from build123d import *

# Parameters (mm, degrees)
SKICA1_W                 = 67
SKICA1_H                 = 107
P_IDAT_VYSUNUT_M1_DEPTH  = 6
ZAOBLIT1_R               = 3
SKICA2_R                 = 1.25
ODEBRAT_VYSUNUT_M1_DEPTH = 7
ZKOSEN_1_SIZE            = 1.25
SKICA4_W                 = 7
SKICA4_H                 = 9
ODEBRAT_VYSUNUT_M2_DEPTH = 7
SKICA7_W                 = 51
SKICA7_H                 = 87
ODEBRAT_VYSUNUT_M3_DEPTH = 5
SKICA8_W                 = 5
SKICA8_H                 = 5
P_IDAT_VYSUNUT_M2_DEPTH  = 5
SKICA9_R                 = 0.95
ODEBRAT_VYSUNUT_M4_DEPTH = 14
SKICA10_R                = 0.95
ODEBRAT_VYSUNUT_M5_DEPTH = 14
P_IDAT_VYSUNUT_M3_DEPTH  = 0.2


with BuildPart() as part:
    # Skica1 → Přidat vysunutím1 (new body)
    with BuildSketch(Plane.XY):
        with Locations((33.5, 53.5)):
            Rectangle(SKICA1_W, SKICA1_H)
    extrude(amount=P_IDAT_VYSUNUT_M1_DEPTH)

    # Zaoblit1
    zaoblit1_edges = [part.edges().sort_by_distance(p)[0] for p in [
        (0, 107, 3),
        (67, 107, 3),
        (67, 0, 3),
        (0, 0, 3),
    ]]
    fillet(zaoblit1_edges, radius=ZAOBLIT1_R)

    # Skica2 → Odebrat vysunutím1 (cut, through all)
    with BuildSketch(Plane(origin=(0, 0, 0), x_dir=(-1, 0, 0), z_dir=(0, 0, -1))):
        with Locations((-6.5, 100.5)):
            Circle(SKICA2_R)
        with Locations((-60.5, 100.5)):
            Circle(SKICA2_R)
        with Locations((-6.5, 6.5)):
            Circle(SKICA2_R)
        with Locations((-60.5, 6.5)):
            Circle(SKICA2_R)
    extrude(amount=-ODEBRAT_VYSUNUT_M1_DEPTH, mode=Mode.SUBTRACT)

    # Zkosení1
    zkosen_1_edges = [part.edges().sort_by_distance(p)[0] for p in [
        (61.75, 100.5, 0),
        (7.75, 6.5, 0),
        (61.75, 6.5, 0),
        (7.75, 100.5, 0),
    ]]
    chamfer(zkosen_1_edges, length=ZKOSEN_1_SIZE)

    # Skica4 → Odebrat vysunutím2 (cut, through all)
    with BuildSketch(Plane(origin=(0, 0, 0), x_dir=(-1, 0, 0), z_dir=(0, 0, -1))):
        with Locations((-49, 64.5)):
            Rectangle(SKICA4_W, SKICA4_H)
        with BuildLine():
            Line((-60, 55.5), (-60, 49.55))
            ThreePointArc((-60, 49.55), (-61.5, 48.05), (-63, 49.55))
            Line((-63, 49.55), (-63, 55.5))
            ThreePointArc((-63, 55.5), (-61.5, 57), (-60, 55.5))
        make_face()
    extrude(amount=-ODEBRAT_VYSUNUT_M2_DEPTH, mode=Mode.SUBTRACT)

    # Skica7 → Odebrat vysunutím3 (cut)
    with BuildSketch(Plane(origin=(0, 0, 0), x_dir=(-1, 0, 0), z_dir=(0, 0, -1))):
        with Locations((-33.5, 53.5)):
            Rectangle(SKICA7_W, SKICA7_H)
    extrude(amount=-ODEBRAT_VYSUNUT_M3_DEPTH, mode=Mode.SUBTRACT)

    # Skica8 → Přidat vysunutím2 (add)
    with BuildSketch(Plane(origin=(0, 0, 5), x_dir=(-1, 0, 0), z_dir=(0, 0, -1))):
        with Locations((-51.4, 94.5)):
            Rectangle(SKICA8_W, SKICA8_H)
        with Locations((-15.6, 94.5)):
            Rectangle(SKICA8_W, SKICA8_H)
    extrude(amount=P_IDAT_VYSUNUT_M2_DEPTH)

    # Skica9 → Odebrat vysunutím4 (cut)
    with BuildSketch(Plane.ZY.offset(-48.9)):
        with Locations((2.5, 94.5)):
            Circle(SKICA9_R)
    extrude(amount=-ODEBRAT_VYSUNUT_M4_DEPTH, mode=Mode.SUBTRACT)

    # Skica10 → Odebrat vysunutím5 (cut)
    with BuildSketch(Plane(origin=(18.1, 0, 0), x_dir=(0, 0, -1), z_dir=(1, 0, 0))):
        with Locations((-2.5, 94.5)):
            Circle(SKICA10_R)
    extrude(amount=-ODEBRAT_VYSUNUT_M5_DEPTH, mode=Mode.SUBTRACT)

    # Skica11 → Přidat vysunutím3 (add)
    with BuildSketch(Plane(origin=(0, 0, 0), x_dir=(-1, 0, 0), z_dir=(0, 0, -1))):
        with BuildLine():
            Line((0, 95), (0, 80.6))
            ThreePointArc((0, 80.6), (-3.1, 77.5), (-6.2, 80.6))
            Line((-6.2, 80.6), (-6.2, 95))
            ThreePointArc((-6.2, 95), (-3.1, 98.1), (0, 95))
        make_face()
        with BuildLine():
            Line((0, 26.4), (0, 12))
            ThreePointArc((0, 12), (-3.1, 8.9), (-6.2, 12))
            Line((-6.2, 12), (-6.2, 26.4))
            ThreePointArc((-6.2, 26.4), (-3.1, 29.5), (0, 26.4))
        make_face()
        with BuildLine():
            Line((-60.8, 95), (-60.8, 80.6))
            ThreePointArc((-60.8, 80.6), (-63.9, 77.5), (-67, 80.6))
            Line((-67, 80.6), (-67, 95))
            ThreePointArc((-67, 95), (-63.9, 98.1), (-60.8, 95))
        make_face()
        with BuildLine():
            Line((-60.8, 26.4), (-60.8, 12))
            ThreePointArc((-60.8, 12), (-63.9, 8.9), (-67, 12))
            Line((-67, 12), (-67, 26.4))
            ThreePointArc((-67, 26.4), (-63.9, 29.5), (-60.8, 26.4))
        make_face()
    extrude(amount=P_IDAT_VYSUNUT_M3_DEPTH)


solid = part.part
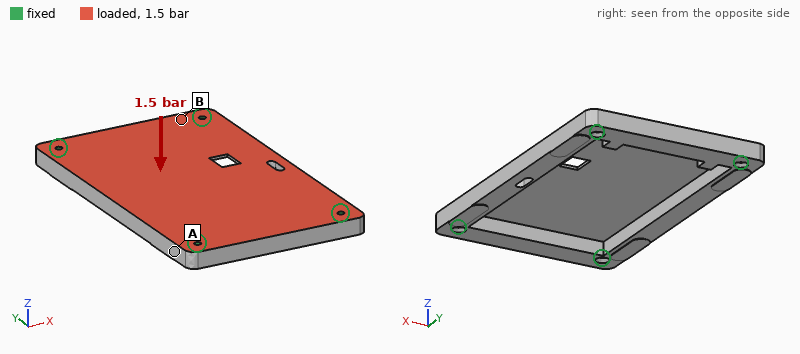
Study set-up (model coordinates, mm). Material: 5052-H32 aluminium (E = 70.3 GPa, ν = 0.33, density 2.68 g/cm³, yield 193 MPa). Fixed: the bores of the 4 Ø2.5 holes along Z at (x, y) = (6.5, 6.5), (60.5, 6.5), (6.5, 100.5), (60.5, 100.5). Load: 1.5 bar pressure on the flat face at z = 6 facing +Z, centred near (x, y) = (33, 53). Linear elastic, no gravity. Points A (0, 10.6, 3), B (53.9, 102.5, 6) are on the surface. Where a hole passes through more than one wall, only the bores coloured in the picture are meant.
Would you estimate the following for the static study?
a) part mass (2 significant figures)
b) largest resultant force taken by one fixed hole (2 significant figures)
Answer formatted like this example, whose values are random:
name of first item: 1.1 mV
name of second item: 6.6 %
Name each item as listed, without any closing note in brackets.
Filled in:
part mass: 56 g
largest resultant force taken by one fixed hole: 300 N
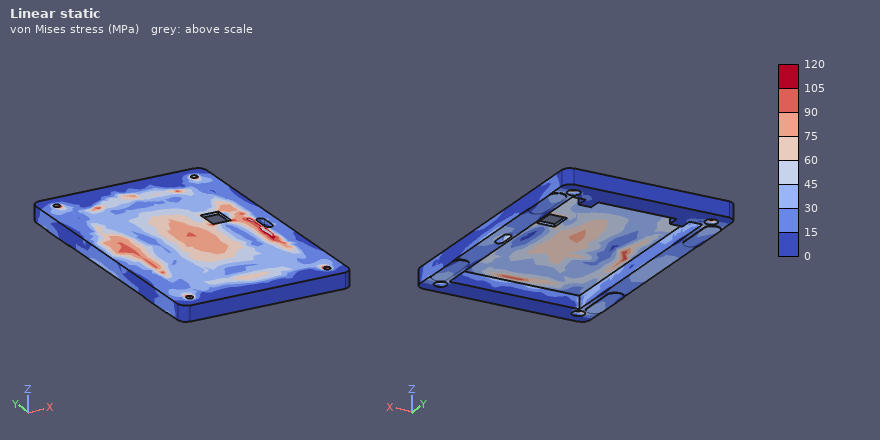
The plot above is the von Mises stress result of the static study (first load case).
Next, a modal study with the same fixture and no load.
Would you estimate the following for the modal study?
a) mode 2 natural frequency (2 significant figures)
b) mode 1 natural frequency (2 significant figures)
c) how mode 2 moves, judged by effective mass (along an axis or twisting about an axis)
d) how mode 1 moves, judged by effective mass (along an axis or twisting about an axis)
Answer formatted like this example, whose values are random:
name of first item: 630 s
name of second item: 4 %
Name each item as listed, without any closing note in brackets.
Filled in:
mode 2 natural frequency: 3200 Hz
mode 1 natural frequency: 2100 Hz
how mode 2 moves, judged by effective mass: twisting about Y
how mode 1 moves, judged by effective mass: along Z
